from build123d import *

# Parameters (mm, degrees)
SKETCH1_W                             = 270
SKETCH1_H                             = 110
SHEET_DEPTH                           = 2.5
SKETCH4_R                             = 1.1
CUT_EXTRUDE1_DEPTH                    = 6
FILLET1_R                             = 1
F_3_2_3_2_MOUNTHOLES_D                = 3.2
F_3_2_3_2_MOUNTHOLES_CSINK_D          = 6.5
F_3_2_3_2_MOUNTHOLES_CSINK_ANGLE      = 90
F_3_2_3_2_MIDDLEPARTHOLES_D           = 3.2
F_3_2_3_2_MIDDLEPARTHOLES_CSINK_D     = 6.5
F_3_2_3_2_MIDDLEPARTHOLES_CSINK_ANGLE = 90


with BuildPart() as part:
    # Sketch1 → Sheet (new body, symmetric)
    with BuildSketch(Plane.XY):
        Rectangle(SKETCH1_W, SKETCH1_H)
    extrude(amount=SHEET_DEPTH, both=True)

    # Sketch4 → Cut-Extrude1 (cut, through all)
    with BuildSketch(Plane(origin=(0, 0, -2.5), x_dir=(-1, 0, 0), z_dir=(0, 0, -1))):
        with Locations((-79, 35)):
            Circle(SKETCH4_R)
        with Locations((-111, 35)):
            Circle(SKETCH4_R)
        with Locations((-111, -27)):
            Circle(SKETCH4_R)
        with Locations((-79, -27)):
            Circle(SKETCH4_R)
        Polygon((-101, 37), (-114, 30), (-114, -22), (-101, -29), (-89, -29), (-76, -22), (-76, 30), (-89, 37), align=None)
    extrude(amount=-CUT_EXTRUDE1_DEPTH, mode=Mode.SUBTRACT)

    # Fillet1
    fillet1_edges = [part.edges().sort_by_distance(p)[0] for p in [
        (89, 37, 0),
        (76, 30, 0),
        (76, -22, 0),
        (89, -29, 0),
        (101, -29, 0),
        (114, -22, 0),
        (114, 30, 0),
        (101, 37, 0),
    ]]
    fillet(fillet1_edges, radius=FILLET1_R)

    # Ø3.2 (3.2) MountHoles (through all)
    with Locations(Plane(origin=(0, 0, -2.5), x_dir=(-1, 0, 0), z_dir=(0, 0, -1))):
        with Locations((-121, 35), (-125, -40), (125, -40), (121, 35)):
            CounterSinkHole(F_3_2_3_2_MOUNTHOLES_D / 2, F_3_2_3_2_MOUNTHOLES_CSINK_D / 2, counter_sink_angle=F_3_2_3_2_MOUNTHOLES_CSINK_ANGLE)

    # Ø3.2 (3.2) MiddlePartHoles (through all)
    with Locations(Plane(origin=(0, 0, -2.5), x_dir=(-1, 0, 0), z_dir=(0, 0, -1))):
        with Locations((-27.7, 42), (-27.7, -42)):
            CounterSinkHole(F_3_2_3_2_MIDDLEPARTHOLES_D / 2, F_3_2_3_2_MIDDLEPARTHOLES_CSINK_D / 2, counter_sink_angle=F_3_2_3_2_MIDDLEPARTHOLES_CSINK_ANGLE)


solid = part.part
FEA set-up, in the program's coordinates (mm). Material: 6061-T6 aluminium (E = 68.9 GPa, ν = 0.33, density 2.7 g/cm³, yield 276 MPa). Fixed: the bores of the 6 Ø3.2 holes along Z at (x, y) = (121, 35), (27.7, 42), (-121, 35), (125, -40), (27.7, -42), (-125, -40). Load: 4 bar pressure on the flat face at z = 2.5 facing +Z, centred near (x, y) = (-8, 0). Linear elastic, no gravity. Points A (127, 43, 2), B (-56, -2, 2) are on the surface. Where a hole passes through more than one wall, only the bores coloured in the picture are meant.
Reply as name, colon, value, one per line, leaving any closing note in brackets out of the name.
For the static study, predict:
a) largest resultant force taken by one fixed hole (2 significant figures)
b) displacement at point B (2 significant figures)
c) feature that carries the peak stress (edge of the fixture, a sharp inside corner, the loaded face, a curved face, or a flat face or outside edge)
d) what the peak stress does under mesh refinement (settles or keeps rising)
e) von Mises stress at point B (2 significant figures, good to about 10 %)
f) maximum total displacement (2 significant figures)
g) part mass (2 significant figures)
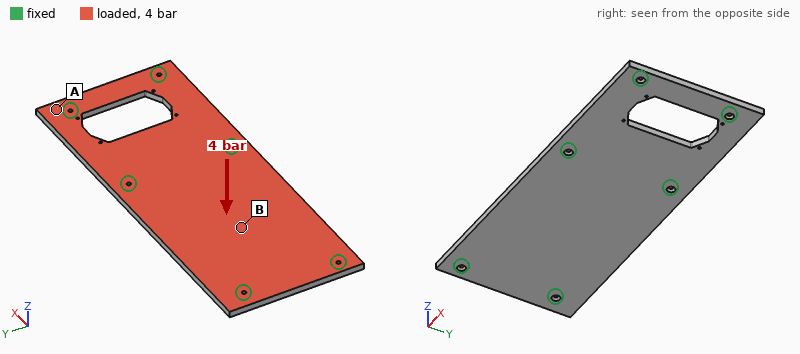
largest resultant force taken by one fixed hole: 3.2 kN
displacement at point B: 1.1 mm
feature that carries the peak stress: edge of the fixture
what the peak stress does under mesh refinement: keeps rising
von Mises stress at point B: 94 MPa
maximum total displacement: 1.2 mm
part mass: 370 g
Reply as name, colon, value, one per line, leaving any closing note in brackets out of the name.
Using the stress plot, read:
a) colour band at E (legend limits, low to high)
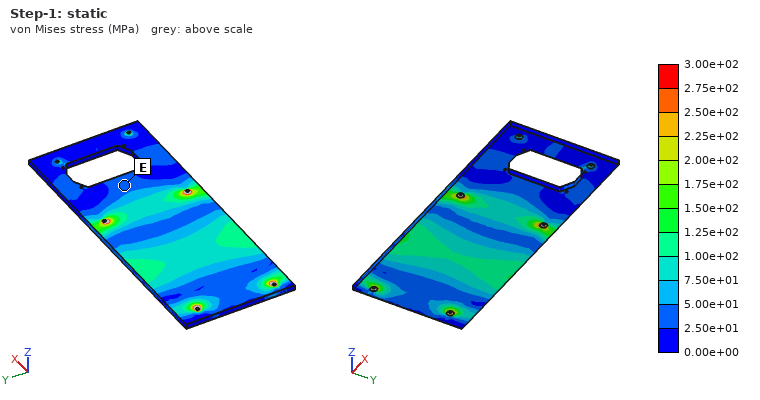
colour band at E: 2.50e+01 to 5.00e+01 MPa
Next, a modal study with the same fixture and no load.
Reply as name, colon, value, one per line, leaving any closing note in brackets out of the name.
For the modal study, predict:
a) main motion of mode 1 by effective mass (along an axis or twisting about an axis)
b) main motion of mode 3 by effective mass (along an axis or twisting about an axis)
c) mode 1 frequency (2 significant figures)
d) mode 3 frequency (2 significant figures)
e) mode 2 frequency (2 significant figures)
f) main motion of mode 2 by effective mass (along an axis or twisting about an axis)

main motion of mode 1 by effective mass: along Z
main motion of mode 3 by effective mass: along Z
mode 1 frequency: 890 Hz
mode 3 frequency: 1900 Hz
mode 2 frequency: 1400 Hz
main motion of mode 2 by effective mass: twisting about X
